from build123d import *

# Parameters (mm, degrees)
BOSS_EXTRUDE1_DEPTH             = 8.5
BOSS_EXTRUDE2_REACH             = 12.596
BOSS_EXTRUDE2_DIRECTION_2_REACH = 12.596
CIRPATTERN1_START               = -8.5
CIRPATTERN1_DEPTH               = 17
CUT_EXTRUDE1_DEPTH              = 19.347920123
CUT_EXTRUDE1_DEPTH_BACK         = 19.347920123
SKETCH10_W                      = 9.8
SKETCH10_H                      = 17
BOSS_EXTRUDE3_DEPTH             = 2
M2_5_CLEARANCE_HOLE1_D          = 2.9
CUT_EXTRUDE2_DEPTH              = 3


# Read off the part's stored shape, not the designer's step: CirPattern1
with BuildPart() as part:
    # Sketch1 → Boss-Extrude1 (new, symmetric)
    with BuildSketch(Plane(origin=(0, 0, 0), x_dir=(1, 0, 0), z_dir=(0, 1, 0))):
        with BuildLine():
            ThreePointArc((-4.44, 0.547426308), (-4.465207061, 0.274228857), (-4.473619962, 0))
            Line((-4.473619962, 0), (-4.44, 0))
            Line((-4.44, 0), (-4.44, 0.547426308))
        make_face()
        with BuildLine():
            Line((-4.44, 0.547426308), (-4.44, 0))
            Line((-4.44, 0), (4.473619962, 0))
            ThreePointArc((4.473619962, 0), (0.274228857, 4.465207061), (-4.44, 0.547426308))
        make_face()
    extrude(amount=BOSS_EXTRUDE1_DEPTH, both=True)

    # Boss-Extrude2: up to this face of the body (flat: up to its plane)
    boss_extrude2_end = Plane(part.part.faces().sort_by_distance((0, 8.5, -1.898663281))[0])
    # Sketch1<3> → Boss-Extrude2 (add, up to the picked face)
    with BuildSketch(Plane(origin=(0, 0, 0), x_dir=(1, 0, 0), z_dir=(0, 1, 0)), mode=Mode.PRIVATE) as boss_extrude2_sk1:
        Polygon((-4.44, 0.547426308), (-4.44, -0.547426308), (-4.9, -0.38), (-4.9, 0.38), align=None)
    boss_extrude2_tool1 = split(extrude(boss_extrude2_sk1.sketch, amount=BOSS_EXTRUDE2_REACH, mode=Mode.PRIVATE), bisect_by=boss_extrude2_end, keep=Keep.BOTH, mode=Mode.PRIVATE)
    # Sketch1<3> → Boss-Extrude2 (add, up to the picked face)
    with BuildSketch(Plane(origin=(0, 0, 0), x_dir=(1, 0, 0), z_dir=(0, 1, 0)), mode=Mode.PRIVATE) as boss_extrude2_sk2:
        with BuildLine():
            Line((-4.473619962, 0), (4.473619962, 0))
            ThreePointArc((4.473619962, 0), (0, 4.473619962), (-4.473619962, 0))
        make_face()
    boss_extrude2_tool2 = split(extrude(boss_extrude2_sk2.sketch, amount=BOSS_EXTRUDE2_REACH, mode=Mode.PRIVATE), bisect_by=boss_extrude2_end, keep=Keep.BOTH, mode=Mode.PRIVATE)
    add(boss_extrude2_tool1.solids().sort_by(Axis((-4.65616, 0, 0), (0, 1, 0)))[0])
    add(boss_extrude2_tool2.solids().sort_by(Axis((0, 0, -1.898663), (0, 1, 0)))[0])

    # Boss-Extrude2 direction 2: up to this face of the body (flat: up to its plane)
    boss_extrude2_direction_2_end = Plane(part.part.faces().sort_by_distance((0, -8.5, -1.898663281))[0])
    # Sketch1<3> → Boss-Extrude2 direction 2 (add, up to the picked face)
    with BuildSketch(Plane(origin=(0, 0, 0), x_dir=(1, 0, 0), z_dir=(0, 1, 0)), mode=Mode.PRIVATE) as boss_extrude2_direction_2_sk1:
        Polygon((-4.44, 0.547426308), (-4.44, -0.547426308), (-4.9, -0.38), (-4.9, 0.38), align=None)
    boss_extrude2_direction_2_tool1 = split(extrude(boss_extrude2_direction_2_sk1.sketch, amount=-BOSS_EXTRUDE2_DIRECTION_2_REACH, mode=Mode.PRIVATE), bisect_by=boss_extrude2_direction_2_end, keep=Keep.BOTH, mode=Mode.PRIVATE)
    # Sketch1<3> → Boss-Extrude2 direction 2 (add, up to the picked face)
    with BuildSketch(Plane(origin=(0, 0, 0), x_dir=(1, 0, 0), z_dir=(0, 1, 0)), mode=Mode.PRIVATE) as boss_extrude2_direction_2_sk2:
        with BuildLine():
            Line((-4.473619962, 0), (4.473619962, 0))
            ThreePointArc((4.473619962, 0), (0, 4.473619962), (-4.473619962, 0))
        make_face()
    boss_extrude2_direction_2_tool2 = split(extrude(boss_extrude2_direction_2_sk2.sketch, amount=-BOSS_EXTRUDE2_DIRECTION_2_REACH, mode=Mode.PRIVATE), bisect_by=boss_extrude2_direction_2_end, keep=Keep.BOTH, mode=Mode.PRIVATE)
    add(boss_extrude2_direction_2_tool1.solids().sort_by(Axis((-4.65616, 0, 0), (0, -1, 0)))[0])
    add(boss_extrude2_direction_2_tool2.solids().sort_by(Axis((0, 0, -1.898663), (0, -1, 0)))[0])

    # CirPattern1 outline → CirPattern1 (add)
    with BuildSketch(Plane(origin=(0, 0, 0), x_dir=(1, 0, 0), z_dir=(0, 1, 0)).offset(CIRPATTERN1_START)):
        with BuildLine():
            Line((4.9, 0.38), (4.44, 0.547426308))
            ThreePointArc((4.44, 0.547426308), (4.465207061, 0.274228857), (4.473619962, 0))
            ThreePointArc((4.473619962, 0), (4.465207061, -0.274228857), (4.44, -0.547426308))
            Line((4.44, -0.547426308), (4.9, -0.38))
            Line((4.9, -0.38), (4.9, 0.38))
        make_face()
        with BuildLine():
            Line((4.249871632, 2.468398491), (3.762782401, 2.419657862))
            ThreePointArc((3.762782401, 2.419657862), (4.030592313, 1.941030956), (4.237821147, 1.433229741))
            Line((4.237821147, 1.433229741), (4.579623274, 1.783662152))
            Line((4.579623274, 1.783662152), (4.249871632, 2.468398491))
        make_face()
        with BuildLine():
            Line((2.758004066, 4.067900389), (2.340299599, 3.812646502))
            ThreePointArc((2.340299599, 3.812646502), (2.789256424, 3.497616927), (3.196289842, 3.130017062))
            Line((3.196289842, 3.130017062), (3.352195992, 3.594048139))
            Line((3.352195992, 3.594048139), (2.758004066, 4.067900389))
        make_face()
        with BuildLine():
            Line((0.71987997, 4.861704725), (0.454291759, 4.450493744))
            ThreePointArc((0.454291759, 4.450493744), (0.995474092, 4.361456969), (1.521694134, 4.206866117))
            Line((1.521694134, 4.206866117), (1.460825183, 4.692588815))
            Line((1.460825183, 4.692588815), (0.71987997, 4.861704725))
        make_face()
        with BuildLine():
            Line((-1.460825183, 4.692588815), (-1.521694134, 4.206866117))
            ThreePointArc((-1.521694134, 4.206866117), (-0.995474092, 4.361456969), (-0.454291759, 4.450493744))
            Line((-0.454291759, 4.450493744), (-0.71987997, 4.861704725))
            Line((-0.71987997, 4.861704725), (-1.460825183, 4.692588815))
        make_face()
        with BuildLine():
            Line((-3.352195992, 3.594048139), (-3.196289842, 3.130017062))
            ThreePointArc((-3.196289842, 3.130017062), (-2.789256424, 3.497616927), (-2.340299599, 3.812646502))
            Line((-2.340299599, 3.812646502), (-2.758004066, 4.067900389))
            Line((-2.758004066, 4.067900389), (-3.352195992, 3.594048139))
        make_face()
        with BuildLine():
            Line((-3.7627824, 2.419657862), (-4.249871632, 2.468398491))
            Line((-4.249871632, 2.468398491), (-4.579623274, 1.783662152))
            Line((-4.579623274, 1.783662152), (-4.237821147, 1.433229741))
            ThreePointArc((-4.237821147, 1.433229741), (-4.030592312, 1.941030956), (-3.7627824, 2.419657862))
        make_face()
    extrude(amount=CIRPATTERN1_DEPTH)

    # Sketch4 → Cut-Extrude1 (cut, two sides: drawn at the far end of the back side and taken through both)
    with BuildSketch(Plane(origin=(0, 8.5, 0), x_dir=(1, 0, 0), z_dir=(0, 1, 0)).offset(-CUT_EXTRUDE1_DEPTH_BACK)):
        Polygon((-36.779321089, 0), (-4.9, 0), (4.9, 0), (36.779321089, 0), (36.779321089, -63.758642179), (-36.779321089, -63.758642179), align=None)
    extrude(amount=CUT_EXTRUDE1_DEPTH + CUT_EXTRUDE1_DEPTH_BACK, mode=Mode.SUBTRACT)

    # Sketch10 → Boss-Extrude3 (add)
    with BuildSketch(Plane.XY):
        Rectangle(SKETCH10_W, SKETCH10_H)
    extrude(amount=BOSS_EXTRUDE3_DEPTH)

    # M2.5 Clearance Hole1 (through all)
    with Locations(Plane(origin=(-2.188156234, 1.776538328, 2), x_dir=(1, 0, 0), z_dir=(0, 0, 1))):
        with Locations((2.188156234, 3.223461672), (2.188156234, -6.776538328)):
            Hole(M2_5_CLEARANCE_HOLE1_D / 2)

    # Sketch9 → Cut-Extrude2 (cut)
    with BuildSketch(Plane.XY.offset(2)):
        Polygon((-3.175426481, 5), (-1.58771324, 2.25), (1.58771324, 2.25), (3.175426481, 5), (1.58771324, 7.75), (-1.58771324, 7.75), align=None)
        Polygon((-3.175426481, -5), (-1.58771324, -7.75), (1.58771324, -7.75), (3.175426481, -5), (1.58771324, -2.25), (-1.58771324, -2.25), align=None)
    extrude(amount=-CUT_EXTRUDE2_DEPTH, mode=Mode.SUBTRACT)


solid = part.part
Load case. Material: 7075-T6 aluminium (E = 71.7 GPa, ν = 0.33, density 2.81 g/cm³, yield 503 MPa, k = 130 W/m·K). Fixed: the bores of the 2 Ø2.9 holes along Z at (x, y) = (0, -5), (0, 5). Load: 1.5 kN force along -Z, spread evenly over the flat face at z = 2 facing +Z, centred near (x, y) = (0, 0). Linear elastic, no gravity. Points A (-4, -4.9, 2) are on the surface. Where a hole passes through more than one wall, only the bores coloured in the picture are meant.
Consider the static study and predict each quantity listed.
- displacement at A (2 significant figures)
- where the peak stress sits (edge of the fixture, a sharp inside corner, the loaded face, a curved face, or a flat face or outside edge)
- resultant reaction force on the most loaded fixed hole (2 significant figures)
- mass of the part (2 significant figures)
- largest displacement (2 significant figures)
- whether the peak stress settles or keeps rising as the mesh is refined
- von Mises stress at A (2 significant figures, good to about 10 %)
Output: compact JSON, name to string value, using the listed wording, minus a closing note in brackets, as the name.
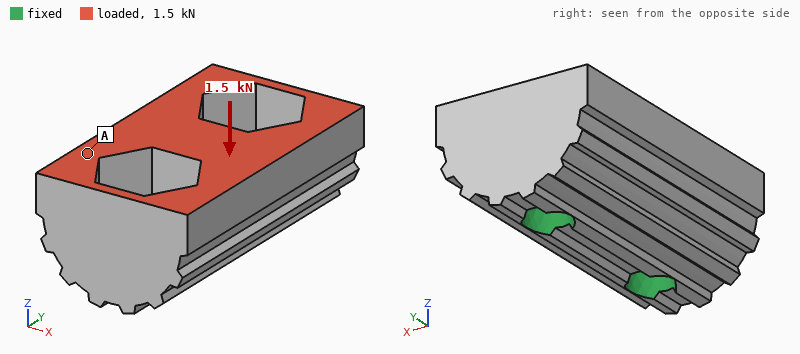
{"displacement at A": "3.3 µm", "where the peak stress sits": "edge of the fixture", "resultant reaction force on the most loaded fixed hole": "760 N", "mass of the part": "2.0 g", "largest displacement": "3.6 µm", "whether the peak stress settles or keeps rising as the mesh is refined": "keeps rising", "von Mises stress at A": "15 MPa"}
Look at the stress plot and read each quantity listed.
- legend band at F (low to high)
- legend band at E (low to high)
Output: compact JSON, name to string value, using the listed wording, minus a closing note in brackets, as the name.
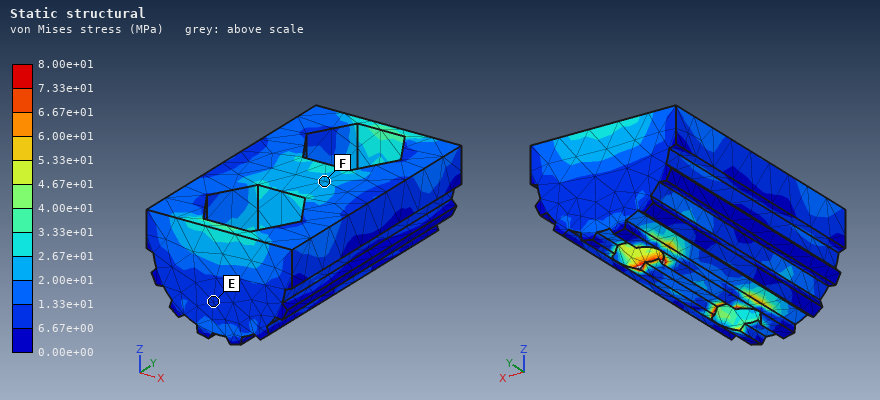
{"legend band at F": "2.00e+01 to 2.67e+01 MPa", "legend band at E": "6.67e+00 to 1.33e+01 MPa"}
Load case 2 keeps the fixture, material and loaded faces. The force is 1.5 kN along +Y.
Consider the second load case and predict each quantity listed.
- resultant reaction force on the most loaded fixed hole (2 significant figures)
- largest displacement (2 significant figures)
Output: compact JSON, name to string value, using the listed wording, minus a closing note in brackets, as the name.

{"resultant reaction force on the most loaded fixed hole": "940 N", "largest displacement": "11 µm"}
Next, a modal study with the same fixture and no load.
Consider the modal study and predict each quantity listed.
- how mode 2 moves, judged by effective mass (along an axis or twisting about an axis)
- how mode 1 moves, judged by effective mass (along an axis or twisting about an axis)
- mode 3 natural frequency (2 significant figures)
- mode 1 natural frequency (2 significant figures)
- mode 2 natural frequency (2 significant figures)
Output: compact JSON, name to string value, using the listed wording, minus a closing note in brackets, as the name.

{"how mode 2 moves, judged by effective mass": "twisting about Z", "how mode 1 moves, judged by effective mass": "along X", "mode 3 natural frequency": "90 kHz", "mode 1 natural frequency": "57 kHz", "mode 2 natural frequency": "80 kHz"}
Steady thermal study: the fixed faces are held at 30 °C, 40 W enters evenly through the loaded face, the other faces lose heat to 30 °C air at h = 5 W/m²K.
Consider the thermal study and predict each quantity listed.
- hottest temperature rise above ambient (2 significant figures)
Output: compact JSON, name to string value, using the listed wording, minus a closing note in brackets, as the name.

{"hottest temperature rise above ambient": "20 K"}
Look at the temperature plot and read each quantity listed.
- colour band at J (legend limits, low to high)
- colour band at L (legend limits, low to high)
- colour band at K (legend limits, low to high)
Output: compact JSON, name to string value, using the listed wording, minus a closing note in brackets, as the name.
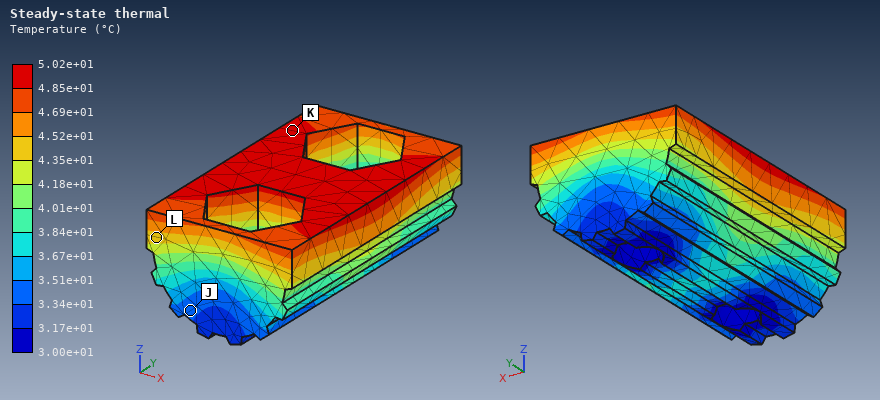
{"colour band at J": "3.34e+01 to 3.51e+01 °C", "colour band at L": "4.35e+01 to 4.52e+01 °C", "colour band at K": "4.85e+01 to 5.02e+01 °C"}
